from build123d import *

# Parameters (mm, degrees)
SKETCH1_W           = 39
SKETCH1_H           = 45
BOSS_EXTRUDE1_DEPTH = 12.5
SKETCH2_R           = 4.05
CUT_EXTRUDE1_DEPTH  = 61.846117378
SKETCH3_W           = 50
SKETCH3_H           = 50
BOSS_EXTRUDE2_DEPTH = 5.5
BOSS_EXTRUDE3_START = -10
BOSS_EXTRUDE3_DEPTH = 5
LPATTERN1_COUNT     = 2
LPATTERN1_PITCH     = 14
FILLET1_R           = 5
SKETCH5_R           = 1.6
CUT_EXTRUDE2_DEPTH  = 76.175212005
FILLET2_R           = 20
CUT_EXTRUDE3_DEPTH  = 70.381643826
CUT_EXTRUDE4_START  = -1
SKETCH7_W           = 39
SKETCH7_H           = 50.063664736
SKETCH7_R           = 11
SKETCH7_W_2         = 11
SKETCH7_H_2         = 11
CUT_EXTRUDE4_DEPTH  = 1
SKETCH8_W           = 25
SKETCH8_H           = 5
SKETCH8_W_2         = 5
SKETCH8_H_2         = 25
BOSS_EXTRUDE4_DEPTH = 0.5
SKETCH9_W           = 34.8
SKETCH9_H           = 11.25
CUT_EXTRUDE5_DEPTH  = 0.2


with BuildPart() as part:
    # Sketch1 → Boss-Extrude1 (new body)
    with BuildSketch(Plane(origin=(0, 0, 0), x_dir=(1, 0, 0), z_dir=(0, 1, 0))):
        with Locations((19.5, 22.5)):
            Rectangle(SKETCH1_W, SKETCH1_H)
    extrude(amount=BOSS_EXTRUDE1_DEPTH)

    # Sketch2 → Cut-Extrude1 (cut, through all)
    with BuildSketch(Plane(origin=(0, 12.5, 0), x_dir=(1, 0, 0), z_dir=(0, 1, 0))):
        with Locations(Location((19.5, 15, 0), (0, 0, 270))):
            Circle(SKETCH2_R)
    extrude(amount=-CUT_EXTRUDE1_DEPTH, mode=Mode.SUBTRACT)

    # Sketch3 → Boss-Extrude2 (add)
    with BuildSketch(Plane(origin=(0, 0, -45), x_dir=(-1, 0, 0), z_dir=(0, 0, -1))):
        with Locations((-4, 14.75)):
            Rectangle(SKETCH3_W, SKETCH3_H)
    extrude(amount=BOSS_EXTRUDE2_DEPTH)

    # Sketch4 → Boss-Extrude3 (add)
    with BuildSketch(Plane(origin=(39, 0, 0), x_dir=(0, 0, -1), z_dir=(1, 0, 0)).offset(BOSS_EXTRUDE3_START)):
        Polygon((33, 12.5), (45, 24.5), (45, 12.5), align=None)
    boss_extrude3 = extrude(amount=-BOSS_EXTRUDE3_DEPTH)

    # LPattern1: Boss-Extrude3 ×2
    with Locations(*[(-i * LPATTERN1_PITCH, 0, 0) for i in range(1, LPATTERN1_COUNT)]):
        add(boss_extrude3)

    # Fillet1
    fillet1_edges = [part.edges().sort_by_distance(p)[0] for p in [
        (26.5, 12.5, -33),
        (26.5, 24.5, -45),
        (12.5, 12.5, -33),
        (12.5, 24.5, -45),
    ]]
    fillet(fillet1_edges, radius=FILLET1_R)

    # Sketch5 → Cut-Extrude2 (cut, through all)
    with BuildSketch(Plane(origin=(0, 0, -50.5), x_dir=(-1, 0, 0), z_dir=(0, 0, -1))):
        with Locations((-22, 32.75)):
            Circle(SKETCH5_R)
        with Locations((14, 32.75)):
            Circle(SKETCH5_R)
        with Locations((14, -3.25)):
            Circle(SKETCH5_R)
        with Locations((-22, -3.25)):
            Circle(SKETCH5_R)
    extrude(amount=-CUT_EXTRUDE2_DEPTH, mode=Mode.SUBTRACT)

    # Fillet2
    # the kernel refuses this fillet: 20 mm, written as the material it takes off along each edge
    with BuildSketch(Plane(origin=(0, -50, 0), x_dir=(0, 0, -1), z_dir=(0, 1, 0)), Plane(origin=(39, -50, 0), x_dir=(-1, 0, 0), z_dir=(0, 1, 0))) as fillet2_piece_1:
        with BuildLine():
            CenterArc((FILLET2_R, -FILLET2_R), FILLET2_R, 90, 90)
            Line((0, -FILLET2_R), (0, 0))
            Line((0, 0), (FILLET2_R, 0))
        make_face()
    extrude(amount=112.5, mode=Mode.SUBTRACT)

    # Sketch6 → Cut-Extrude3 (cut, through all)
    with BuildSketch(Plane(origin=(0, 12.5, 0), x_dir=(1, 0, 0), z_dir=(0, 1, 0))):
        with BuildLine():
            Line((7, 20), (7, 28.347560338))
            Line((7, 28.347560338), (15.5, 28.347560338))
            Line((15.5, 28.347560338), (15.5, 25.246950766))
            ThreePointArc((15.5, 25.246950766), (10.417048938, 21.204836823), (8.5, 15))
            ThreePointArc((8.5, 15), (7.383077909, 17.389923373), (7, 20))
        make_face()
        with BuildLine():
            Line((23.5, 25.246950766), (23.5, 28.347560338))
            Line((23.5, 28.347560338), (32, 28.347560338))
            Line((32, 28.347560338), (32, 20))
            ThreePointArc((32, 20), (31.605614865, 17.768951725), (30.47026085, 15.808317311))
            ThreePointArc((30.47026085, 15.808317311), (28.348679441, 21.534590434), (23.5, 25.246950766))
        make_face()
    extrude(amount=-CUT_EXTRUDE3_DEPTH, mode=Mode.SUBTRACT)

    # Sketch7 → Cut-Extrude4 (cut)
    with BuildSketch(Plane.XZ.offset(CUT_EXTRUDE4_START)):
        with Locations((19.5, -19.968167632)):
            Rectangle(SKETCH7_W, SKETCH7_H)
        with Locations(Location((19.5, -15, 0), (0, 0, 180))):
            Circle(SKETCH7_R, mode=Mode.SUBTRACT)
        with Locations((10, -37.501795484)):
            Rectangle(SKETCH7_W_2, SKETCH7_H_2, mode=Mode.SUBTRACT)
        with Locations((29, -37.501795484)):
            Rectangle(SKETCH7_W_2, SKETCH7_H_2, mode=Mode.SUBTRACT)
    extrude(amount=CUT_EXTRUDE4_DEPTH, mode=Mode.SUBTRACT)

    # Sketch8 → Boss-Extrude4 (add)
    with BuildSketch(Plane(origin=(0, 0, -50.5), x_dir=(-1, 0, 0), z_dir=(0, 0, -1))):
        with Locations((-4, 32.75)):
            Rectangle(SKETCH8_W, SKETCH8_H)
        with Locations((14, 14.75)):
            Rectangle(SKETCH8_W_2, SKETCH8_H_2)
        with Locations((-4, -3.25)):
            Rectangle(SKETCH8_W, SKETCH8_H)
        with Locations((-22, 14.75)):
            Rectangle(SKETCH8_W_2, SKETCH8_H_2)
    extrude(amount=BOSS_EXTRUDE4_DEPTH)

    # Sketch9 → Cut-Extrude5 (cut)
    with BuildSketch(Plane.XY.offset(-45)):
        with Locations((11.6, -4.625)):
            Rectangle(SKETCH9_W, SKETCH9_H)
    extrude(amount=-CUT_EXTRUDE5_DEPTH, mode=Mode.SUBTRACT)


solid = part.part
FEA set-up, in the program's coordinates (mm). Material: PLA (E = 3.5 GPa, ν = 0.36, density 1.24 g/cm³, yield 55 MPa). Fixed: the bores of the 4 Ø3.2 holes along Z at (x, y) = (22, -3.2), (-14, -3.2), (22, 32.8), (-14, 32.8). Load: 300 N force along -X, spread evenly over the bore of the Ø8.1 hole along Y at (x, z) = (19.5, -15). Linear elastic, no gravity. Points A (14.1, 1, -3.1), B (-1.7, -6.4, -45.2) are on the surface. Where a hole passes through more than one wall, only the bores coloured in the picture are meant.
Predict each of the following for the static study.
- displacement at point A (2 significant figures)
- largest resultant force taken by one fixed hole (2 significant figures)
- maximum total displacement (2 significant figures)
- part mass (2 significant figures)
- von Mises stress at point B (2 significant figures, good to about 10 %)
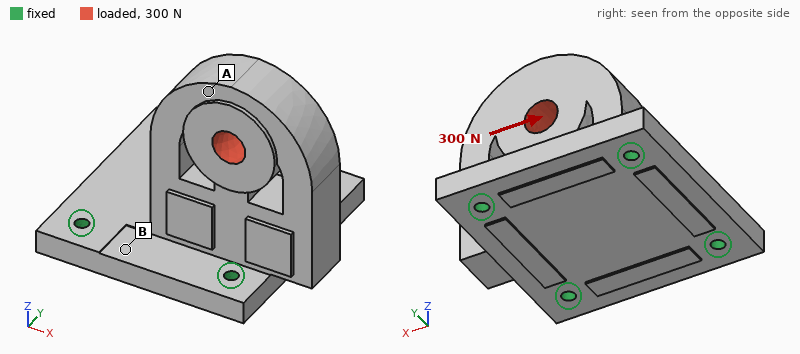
0.39 mm
240 N
0.41 mm
39 g
5.9 MPa
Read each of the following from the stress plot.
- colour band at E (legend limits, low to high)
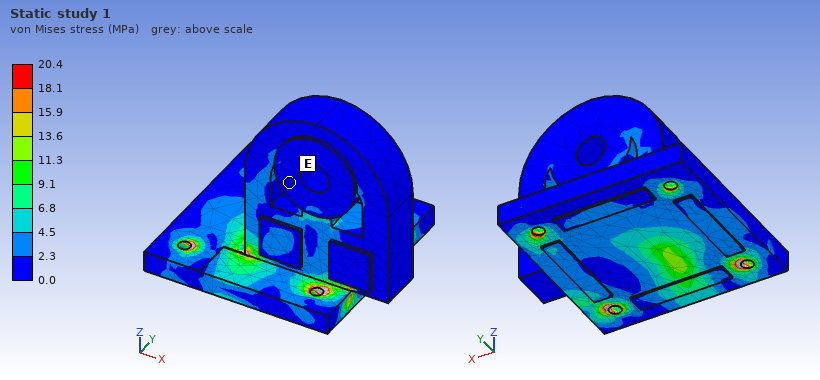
0.0 to 2.3 MPa
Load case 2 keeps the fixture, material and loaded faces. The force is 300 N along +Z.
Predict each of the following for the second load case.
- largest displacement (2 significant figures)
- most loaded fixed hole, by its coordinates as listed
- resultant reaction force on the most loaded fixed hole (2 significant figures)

50 µm
(22, -3.2)
210 N
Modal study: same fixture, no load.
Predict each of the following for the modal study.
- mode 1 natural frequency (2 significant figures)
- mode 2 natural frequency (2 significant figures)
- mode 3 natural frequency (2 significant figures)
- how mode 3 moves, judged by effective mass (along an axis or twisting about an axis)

1300 Hz
1300 Hz
3200 Hz
along Z
